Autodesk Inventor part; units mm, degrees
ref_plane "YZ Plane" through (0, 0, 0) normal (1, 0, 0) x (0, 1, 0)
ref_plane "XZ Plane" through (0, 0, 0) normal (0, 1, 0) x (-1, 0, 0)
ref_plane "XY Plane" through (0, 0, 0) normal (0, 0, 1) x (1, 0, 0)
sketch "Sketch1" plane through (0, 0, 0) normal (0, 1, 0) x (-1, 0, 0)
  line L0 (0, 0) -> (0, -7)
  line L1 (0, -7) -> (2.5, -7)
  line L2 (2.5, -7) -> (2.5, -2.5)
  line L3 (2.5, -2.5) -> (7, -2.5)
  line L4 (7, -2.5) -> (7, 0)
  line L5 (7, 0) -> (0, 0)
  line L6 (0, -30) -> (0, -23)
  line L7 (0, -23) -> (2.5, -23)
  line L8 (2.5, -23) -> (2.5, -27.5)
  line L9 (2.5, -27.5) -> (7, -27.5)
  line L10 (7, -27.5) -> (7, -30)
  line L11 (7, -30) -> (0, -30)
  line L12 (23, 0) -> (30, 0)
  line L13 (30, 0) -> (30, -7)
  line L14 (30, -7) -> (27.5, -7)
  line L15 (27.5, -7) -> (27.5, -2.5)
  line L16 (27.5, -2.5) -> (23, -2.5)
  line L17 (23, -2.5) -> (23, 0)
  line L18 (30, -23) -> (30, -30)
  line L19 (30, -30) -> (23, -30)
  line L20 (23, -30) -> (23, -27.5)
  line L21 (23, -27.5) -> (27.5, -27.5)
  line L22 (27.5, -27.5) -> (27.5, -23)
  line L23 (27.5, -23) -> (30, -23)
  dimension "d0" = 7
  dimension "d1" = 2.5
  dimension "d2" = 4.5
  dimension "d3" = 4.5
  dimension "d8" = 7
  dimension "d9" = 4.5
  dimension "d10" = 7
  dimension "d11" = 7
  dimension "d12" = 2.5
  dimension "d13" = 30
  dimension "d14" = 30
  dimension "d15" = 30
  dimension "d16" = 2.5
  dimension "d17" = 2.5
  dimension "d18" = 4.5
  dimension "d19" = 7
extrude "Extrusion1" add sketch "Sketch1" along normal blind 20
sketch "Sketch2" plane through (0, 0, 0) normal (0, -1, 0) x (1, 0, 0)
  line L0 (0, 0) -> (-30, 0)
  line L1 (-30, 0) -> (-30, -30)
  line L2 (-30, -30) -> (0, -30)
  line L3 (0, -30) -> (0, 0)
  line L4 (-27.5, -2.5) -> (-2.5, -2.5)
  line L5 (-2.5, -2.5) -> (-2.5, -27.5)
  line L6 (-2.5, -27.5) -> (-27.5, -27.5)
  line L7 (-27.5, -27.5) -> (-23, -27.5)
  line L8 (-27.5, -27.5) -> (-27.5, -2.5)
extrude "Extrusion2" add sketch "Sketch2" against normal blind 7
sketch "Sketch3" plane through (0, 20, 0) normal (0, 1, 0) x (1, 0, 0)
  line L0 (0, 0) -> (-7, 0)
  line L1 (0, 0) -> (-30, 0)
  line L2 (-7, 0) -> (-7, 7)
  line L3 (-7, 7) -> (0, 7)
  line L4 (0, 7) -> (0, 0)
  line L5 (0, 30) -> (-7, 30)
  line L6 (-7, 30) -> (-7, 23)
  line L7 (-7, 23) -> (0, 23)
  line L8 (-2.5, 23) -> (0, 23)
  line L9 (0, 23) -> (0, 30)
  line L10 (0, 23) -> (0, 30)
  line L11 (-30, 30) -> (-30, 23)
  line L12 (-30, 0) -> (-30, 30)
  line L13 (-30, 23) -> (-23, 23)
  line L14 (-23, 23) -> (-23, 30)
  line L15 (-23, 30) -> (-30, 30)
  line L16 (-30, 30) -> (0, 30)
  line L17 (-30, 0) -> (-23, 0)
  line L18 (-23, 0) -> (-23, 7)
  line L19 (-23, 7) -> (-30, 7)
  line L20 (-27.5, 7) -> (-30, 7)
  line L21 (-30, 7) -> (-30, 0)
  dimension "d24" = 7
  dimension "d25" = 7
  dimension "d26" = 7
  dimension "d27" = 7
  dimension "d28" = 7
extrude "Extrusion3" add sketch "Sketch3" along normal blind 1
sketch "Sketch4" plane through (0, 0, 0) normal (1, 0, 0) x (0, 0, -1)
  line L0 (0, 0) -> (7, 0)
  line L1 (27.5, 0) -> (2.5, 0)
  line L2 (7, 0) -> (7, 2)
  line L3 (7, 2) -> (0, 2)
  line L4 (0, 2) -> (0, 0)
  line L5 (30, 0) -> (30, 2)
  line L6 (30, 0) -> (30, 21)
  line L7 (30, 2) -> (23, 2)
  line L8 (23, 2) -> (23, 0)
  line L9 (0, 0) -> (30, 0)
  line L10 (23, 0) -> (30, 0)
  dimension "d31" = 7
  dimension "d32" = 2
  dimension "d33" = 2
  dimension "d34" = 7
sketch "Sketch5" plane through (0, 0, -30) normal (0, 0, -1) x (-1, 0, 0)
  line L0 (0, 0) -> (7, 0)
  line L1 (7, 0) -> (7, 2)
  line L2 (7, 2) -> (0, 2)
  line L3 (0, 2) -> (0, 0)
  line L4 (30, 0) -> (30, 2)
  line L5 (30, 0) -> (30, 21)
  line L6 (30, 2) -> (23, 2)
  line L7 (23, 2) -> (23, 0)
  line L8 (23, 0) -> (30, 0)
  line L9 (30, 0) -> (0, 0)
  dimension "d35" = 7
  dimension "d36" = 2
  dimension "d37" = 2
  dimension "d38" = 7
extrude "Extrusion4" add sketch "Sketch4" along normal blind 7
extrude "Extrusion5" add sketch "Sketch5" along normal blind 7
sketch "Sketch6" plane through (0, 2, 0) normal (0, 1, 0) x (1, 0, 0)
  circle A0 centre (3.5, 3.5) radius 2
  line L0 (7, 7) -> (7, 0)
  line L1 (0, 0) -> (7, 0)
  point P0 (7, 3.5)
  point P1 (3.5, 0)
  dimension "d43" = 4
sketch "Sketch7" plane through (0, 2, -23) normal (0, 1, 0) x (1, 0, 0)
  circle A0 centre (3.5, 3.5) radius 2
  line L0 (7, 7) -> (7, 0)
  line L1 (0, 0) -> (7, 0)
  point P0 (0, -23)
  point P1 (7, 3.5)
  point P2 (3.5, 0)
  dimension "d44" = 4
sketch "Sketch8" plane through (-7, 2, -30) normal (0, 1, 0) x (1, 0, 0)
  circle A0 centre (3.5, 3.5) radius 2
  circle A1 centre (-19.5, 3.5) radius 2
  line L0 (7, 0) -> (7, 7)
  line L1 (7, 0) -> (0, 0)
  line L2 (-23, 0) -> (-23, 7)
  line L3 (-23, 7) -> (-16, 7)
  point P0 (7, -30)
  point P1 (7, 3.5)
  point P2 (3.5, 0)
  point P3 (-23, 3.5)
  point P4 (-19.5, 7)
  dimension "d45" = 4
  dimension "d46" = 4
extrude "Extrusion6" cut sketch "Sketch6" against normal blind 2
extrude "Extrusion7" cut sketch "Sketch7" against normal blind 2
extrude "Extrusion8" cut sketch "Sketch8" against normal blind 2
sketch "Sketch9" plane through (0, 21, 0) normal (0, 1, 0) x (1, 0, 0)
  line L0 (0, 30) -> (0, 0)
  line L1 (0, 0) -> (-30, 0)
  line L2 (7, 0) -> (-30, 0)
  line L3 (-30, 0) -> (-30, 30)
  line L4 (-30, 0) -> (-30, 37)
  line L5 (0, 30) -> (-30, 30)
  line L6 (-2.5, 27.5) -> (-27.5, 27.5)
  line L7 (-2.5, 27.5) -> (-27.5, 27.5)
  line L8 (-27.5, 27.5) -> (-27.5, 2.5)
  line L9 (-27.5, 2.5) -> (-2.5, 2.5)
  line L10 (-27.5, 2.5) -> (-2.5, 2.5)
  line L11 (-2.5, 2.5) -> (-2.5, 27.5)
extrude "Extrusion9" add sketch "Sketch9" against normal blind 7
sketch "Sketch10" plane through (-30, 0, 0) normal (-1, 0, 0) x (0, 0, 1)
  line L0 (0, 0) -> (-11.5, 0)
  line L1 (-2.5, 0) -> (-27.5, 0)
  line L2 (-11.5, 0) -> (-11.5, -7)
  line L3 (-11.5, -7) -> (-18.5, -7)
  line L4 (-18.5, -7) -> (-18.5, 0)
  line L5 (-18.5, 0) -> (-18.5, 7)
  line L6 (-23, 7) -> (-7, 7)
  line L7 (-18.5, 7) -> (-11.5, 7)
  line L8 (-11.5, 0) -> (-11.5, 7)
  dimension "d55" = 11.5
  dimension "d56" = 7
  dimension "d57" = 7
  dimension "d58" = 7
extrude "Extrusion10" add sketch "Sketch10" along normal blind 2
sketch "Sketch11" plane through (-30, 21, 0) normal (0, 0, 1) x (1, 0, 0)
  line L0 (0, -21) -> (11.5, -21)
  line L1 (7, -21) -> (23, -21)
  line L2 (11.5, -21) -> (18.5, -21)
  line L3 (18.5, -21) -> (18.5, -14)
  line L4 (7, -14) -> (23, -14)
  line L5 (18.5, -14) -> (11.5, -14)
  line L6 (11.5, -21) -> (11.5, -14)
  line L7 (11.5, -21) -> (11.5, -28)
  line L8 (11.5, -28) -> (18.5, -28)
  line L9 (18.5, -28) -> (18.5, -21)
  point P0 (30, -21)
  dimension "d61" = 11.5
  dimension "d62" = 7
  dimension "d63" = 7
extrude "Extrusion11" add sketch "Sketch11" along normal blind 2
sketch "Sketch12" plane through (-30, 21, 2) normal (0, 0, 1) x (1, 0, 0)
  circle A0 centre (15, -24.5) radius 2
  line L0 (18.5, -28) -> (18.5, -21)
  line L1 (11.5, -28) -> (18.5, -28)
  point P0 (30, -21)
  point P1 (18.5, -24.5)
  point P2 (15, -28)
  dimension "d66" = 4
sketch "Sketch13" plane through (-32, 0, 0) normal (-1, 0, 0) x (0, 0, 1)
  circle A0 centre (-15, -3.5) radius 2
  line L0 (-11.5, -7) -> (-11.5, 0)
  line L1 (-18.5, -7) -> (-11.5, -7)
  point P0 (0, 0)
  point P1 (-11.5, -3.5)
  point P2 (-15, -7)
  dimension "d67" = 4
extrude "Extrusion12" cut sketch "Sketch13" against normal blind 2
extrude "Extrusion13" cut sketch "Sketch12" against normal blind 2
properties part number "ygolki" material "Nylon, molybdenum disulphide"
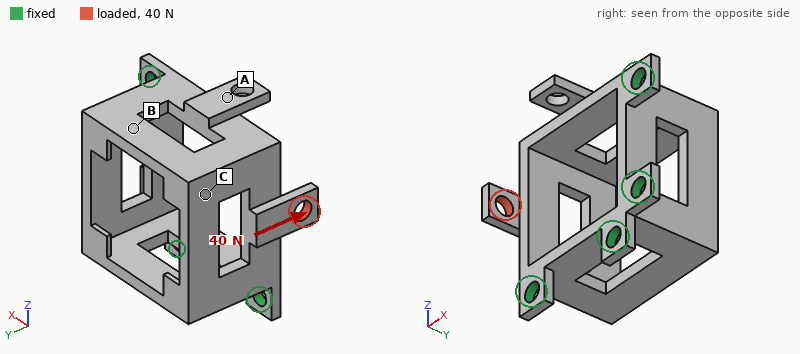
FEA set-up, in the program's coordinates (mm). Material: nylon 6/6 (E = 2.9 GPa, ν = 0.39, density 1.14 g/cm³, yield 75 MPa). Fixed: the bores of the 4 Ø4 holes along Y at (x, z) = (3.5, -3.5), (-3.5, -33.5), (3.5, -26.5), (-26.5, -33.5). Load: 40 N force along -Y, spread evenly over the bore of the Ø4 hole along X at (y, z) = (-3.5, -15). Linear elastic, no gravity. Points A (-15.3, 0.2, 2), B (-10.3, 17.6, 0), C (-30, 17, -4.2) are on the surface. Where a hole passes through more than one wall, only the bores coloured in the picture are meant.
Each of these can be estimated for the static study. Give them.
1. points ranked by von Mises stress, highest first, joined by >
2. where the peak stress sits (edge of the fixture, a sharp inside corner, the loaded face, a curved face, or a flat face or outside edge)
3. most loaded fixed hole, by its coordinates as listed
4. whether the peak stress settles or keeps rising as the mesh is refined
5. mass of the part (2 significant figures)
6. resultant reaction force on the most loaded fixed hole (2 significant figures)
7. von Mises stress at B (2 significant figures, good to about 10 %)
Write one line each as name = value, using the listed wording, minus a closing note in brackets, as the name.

points ranked by von Mises stress, highest first, joined by > = B > C > A
where the peak stress sits = edge of the fixture
most loaded fixed hole, by its coordinates as listed = (-26.5, -33.5)
whether the peak stress settles or keeps rising as the mesh is refined = keeps rising
mass of the part = 6.1 g
resultant reaction force on the most loaded fixed hole = 45 N
von Mises stress at B = 5.6 MPa
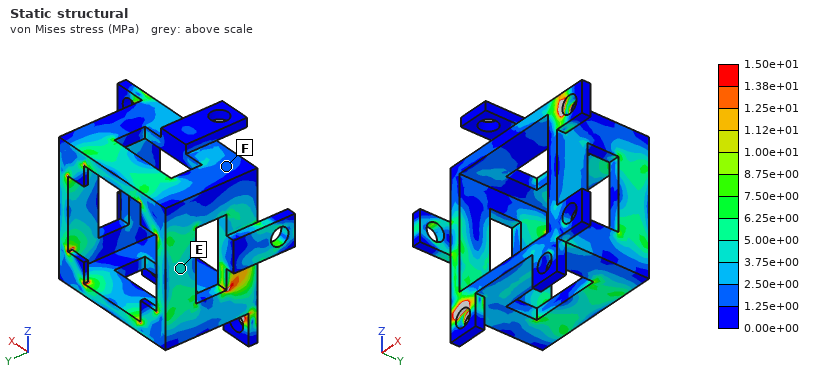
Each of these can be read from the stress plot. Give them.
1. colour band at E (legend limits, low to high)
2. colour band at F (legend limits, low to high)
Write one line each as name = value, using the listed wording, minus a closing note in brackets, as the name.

colour band at E = 3.75e+00 to 5.00e+00 MPa
colour band at F = 1.25e+00 to 2.50e+00 MPa
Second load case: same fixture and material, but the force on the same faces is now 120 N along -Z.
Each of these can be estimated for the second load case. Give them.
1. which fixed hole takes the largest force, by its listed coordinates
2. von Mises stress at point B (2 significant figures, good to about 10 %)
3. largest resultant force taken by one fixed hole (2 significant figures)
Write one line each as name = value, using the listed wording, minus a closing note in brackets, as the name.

which fixed hole takes the largest force, by its listed coordinates = (-26.5, -33.5)
von Mises stress at point B = 5.7 MPa
largest resultant force taken by one fixed hole = 130 N
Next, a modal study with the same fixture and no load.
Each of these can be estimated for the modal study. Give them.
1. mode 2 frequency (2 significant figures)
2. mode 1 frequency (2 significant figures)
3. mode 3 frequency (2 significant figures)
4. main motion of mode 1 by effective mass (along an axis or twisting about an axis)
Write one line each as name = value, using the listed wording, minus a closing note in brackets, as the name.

mode 2 frequency = 2500 Hz
mode 1 frequency = 820 Hz
mode 3 frequency = 3200 Hz
main motion of mode 1 by effective mass = along Y
